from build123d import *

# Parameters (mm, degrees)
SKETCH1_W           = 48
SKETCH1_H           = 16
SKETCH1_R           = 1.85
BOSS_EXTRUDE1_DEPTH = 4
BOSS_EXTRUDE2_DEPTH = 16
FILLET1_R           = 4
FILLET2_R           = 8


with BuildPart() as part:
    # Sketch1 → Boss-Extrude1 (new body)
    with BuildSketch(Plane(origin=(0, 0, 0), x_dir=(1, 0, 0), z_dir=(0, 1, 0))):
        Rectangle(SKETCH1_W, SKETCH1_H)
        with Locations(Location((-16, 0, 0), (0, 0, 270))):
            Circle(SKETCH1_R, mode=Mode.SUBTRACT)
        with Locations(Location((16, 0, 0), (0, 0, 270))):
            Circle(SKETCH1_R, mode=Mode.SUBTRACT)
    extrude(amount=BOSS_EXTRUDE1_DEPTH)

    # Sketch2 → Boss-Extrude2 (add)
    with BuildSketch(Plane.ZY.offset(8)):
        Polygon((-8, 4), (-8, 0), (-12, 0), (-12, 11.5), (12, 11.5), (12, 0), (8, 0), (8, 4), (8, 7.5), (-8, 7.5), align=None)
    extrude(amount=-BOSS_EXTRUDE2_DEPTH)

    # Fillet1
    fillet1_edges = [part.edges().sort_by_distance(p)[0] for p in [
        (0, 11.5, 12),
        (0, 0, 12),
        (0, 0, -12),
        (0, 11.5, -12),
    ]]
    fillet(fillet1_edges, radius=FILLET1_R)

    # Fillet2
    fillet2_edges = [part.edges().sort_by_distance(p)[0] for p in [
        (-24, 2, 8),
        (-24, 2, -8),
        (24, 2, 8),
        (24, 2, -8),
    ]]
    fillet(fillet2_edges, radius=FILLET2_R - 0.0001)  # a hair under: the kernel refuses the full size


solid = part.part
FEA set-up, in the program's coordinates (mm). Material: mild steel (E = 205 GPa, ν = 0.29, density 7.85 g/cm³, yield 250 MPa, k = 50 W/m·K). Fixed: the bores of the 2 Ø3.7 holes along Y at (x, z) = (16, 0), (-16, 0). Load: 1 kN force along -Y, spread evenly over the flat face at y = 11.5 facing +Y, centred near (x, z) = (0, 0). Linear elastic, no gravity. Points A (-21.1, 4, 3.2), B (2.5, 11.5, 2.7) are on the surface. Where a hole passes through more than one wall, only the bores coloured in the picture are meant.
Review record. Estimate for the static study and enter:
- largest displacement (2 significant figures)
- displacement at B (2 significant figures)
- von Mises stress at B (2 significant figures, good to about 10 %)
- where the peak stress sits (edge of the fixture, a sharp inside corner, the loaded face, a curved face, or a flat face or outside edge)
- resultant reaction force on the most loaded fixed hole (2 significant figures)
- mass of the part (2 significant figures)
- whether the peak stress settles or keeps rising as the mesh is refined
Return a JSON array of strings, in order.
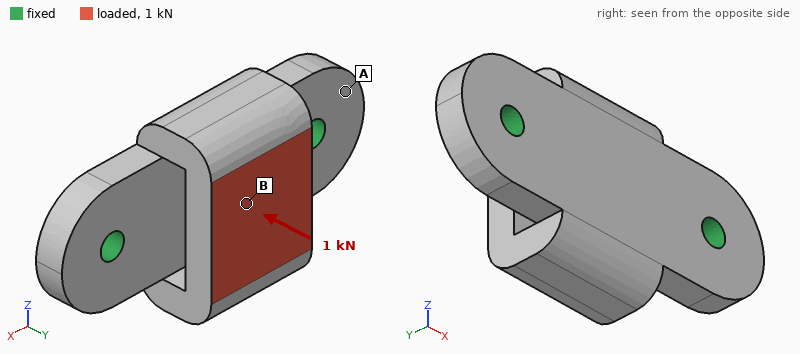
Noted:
["11 µm", "10 µm", "22 MPa", "edge of the fixture", "500 N", "40 g", "keeps rising"]
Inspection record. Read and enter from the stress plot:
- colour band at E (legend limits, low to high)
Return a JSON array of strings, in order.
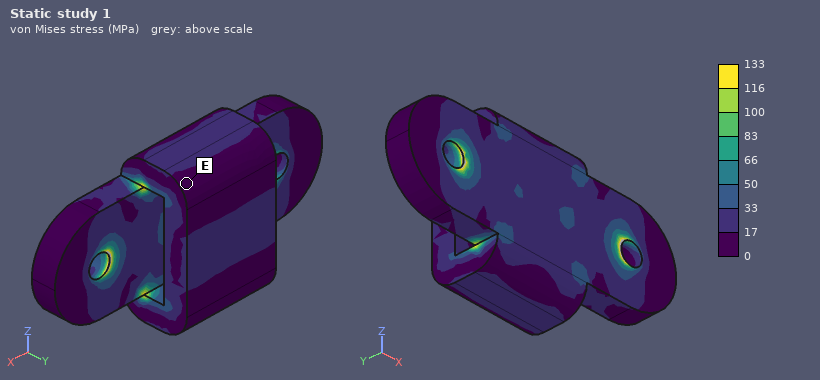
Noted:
["0 to 17 MPa"]
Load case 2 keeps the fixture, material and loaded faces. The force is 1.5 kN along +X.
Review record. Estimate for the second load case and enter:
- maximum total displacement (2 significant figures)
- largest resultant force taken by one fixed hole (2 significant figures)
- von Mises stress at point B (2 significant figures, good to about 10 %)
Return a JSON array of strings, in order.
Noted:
["17 µm", "960 N", "21 MPa"]
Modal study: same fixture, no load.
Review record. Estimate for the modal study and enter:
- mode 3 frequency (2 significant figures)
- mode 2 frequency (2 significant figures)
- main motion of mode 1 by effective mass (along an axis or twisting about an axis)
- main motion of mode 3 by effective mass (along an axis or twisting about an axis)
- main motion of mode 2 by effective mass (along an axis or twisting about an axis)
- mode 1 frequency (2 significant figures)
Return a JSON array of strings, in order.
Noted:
["16 kHz", "12 kHz", "along Z", "along X", "along Y", "7900 Hz"]
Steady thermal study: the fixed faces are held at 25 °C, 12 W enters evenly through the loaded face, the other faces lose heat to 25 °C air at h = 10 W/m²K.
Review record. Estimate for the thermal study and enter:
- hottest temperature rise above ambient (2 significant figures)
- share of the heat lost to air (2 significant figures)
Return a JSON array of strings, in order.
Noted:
["47 K", "4.8 %"]
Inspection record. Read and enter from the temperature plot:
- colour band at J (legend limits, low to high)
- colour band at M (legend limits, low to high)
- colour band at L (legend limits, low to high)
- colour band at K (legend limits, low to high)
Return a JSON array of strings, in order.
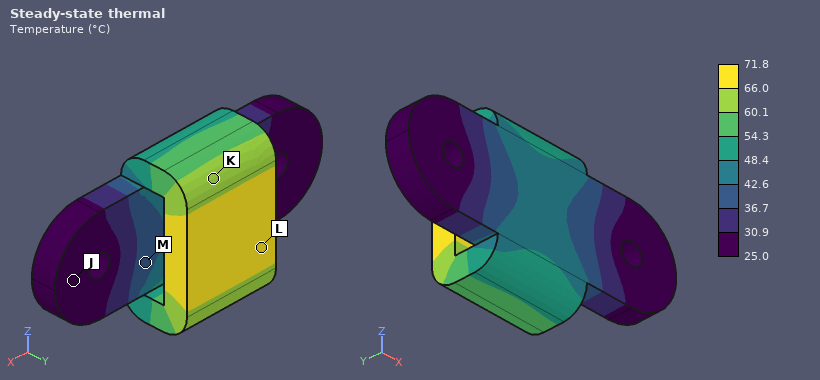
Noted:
["25.0 to 30.9 °C", "36.7 to 42.6 °C", "66.0 to 71.8 °C", "60.1 to 66.0 °C"]
